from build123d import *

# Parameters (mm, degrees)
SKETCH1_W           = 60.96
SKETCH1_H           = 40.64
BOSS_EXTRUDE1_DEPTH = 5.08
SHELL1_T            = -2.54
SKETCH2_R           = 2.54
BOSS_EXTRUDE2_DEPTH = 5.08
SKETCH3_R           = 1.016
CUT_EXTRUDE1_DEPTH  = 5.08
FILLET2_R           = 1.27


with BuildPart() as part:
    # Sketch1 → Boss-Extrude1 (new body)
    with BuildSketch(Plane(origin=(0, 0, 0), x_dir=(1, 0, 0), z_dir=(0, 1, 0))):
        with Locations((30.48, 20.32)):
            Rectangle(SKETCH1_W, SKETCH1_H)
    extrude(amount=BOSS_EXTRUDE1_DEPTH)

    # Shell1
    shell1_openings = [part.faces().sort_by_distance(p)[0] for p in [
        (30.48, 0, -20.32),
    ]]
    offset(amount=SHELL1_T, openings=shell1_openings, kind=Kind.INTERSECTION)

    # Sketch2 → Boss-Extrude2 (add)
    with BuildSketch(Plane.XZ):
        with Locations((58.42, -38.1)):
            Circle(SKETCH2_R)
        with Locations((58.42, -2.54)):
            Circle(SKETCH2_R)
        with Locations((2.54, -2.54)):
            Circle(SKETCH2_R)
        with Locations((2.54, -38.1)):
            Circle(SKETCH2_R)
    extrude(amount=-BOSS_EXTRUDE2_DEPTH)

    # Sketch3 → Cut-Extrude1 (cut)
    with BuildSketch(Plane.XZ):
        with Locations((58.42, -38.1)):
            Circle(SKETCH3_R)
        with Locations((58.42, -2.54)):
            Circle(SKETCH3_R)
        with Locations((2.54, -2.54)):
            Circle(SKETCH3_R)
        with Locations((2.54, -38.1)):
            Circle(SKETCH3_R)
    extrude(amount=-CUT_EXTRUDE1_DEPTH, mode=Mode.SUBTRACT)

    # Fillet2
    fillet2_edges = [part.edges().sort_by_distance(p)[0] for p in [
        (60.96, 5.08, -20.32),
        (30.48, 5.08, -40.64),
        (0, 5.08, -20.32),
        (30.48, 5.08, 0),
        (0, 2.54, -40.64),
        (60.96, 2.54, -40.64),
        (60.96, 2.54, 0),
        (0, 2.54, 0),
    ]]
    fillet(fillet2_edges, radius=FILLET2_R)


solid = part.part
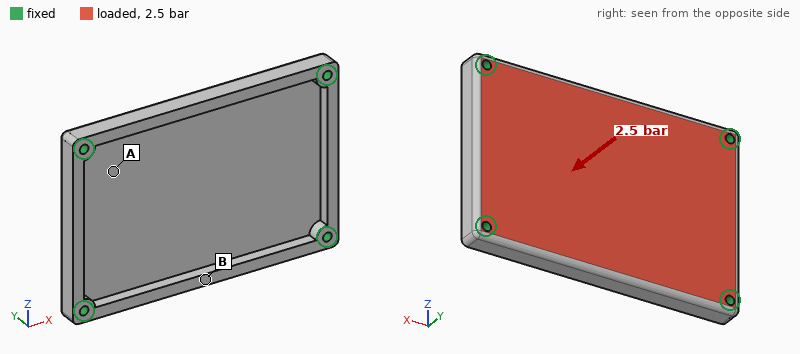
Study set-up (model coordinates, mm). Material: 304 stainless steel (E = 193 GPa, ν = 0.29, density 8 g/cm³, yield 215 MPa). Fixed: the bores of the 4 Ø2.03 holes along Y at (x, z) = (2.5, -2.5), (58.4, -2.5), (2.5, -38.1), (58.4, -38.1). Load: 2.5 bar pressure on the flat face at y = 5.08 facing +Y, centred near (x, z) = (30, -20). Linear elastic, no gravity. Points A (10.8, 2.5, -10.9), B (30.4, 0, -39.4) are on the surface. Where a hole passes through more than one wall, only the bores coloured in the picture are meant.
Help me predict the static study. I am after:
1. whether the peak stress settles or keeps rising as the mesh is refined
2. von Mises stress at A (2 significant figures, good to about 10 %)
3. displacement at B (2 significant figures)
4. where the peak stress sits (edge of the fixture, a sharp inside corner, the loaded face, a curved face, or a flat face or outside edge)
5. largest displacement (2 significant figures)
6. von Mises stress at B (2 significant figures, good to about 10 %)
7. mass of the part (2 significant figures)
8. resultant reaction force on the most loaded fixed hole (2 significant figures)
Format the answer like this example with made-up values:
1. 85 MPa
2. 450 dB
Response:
1. keeps rising
2. 8.6 MPa
3. 11 µm
4. edge of the fixture
5. 19 µm
6. 32 MPa
7. 60 g
8. 160 N
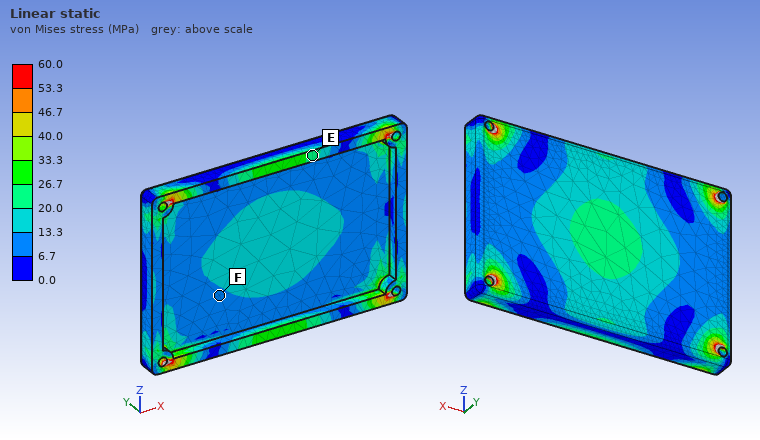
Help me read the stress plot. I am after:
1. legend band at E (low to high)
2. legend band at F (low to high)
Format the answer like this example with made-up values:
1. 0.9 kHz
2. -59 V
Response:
1. 20.0 to 26.7 MPa
2. 6.7 to 13.3 MPa
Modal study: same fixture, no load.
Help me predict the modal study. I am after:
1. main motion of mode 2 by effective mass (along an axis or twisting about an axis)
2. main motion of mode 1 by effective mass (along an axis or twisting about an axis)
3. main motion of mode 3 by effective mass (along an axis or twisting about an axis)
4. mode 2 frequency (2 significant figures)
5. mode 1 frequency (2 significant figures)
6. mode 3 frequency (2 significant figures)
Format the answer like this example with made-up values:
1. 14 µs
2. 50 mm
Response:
1. twisting about X
2. along Y
3. twisting about Z
4. 7400 Hz
5. 4700 Hz
6. 10 kHz
